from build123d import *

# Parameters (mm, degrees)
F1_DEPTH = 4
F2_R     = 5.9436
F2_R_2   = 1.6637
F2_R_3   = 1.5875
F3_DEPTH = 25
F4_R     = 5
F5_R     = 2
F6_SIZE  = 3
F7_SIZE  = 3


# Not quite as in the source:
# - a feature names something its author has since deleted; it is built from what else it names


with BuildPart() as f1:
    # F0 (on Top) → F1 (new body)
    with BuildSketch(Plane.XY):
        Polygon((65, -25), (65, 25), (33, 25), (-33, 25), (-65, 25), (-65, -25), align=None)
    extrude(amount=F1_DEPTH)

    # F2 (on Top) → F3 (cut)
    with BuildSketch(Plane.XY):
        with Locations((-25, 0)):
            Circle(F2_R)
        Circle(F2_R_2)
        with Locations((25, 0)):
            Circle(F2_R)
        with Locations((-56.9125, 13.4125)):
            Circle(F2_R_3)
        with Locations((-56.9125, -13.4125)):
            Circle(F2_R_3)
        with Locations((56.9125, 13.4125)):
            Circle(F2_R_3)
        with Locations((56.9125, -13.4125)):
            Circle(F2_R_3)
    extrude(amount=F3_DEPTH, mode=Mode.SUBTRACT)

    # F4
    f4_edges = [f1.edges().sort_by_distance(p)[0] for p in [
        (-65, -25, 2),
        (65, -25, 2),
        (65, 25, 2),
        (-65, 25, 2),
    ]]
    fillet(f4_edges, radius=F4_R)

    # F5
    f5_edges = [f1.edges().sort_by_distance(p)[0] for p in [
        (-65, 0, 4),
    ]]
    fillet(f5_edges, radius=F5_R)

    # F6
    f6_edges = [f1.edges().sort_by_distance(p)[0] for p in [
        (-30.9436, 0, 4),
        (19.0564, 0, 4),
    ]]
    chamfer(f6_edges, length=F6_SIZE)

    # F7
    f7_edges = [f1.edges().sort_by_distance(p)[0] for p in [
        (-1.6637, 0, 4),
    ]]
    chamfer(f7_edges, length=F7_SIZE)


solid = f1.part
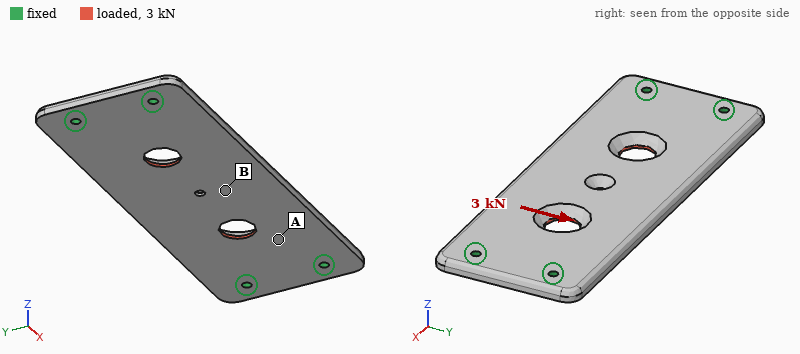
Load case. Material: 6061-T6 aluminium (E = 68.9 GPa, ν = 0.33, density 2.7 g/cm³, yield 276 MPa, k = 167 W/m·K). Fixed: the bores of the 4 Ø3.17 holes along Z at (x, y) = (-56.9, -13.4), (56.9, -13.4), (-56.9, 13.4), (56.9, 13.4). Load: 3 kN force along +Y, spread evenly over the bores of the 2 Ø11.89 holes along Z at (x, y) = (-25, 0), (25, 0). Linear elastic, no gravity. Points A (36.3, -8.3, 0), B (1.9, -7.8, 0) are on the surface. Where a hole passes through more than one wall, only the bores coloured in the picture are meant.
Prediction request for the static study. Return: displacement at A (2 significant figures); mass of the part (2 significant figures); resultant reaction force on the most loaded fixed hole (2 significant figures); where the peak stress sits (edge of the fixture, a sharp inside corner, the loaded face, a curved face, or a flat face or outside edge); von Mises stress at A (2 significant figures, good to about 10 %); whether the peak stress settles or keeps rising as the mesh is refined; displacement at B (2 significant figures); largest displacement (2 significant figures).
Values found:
16 µm
65 g
1.2 kN
edge of the fixture
26 MPa
keeps rising
32 µm
55 µm
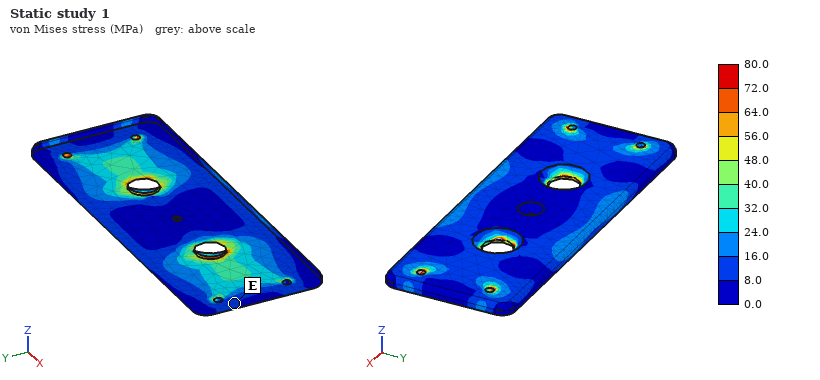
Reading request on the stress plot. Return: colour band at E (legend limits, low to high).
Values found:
8.0 to 16.0 MPa
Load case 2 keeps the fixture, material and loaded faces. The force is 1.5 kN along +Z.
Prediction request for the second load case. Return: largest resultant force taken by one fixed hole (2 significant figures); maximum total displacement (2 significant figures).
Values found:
390 N
0.44 mm
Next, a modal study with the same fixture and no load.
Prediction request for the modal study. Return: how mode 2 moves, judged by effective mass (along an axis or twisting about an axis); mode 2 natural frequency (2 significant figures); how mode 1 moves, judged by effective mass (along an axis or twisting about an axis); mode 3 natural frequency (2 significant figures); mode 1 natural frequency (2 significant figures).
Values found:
twisting about X
2600 Hz
along Z
4100 Hz
1600 Hz
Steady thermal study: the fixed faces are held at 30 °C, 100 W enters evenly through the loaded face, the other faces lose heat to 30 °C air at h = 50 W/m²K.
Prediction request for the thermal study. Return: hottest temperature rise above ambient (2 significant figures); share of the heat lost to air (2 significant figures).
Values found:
65 K
20 %
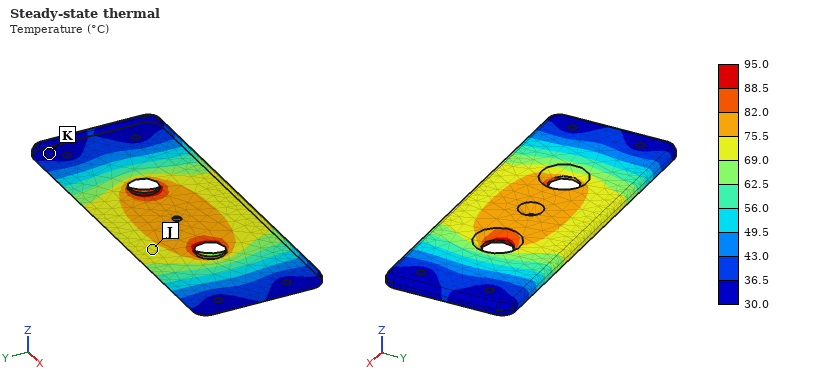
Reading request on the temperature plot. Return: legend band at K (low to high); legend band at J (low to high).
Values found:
30.0 to 36.5 °C
69.0 to 75.5 °C
